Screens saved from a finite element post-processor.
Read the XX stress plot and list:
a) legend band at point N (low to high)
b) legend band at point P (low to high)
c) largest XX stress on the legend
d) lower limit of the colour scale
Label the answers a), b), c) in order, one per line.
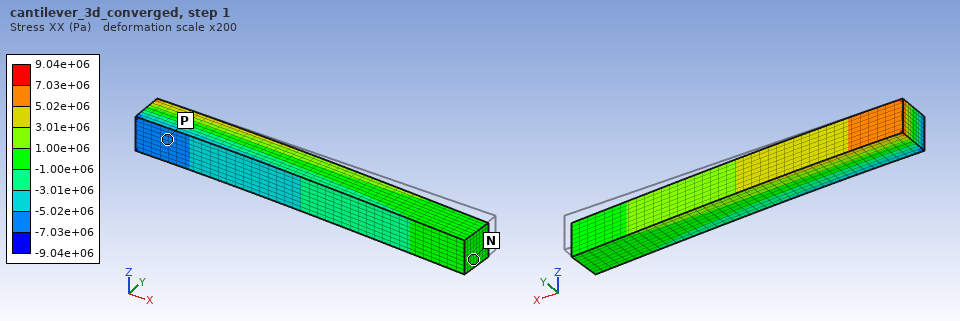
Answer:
a) -1.00e+06 to 1.00e+06 Pa
b) -7.03e+06 to -5.02e+06 Pa
c) 9.04e+06 Pa
d) -9.04e+06 Pa
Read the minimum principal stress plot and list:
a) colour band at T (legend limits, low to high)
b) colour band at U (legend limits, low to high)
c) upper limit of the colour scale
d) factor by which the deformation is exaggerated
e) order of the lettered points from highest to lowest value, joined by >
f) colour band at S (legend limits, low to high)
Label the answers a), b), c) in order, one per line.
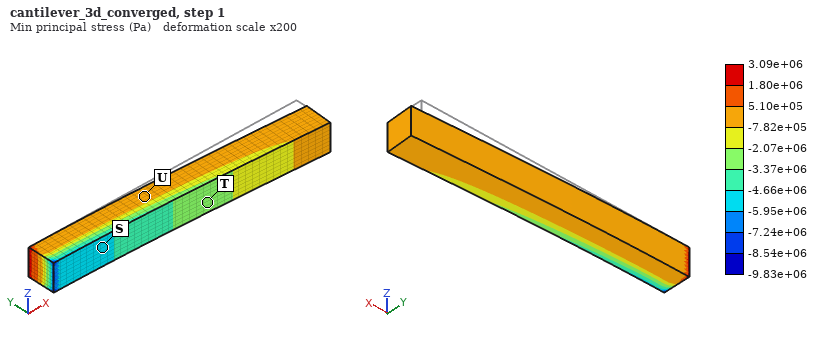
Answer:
a) -3.37e+06 to -2.07e+06 Pa
b) -7.82e+05 to 5.10e+05 Pa
c) 3.09e+06 Pa
d) 200
e) U > T > S
f) -5.95e+06 to -4.66e+06 Pa
